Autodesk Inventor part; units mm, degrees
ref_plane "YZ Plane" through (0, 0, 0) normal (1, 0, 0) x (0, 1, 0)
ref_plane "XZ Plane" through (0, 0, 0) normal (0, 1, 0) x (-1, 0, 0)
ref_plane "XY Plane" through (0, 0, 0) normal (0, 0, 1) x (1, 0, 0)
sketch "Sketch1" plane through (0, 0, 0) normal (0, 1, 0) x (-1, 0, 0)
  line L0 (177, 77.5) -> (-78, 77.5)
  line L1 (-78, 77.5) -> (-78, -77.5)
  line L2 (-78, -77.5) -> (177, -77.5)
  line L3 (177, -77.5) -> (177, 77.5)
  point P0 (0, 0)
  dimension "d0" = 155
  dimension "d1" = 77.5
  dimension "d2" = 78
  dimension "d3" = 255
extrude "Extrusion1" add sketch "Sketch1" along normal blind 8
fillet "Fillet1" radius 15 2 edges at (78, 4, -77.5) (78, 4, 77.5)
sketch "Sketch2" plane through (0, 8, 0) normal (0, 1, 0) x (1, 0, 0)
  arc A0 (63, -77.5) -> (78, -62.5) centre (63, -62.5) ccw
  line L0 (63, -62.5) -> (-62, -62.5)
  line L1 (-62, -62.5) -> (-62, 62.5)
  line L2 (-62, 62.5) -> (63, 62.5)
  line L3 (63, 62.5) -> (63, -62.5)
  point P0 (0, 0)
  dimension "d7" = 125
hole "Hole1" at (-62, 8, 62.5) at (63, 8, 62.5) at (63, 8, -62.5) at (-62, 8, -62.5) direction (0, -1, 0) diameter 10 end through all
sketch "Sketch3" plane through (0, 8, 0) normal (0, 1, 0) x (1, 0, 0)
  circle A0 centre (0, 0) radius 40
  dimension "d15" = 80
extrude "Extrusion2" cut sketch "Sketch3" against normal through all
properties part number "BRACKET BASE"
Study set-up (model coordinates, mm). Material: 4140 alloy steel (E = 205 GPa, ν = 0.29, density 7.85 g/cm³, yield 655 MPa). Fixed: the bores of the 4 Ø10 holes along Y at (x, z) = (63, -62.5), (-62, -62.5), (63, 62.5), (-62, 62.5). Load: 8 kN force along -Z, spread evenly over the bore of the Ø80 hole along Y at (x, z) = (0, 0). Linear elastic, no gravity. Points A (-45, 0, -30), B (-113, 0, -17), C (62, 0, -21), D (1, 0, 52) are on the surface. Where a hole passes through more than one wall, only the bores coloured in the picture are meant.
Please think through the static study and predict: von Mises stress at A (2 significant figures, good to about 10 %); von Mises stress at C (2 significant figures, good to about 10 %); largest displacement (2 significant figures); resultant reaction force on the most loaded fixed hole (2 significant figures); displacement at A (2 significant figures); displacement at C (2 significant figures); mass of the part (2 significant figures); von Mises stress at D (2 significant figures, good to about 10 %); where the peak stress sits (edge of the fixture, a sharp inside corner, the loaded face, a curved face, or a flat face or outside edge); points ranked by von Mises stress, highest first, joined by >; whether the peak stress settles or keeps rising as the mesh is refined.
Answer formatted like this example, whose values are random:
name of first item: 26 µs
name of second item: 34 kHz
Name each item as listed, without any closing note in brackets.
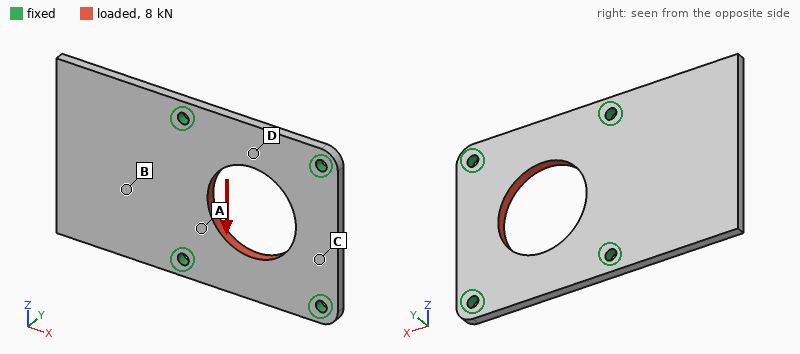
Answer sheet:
von Mises stress at A: 6.3 MPa
von Mises stress at C: 4.7 MPa
largest displacement: 3.5 µm
resultant reaction force on the most loaded fixed hole: 2.2 kN
displacement at A: 1.4 µm
displacement at C: 1.1 µm
mass of the part: 2.1 kg
von Mises stress at D: 2.7 MPa
where the peak stress sits: edge of the fixture
points ranked by von Mises stress, highest first, joined by >: A > C > D > B
whether the peak stress settles or keeps rising as the mesh is refined: keeps rising
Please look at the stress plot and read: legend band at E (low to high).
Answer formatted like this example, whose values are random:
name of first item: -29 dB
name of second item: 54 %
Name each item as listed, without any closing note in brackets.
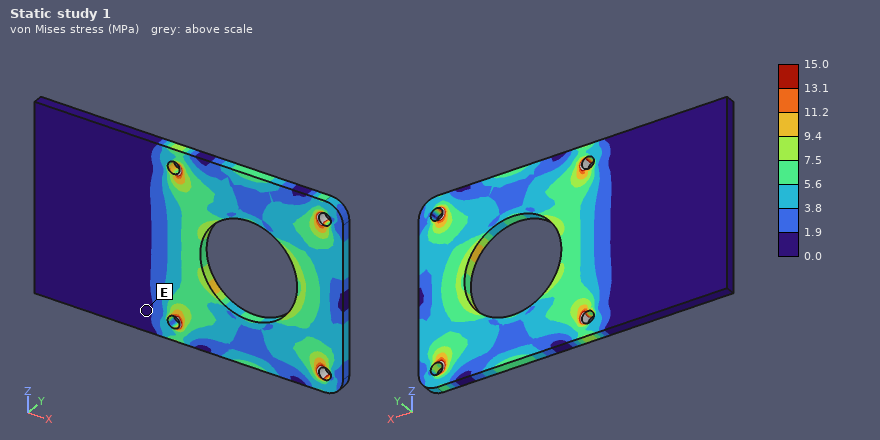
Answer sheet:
legend band at E: 0.0 to 1.9 MPa
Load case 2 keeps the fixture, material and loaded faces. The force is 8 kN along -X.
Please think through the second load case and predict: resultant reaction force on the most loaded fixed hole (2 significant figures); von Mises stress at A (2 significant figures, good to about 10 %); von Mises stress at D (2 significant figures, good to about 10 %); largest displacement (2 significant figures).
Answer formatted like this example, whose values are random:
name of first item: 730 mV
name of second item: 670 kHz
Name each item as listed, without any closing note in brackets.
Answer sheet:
resultant reaction force on the most loaded fixed hole: 2.2 kN
von Mises stress at A: 3.6 MPa
von Mises stress at D: 5.8 MPa
largest displacement: 4.0 µm
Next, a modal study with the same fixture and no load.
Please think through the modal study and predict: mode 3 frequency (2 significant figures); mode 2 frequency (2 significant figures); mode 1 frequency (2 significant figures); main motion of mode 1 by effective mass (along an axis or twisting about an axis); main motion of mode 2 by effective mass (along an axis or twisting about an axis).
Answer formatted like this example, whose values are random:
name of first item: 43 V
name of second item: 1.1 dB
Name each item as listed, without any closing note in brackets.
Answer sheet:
mode 3 frequency: 2200 Hz
mode 2 frequency: 1000 Hz
mode 1 frequency: 440 Hz
main motion of mode 1 by effective mass: along Y
main motion of mode 2 by effective mass: twisting about X
